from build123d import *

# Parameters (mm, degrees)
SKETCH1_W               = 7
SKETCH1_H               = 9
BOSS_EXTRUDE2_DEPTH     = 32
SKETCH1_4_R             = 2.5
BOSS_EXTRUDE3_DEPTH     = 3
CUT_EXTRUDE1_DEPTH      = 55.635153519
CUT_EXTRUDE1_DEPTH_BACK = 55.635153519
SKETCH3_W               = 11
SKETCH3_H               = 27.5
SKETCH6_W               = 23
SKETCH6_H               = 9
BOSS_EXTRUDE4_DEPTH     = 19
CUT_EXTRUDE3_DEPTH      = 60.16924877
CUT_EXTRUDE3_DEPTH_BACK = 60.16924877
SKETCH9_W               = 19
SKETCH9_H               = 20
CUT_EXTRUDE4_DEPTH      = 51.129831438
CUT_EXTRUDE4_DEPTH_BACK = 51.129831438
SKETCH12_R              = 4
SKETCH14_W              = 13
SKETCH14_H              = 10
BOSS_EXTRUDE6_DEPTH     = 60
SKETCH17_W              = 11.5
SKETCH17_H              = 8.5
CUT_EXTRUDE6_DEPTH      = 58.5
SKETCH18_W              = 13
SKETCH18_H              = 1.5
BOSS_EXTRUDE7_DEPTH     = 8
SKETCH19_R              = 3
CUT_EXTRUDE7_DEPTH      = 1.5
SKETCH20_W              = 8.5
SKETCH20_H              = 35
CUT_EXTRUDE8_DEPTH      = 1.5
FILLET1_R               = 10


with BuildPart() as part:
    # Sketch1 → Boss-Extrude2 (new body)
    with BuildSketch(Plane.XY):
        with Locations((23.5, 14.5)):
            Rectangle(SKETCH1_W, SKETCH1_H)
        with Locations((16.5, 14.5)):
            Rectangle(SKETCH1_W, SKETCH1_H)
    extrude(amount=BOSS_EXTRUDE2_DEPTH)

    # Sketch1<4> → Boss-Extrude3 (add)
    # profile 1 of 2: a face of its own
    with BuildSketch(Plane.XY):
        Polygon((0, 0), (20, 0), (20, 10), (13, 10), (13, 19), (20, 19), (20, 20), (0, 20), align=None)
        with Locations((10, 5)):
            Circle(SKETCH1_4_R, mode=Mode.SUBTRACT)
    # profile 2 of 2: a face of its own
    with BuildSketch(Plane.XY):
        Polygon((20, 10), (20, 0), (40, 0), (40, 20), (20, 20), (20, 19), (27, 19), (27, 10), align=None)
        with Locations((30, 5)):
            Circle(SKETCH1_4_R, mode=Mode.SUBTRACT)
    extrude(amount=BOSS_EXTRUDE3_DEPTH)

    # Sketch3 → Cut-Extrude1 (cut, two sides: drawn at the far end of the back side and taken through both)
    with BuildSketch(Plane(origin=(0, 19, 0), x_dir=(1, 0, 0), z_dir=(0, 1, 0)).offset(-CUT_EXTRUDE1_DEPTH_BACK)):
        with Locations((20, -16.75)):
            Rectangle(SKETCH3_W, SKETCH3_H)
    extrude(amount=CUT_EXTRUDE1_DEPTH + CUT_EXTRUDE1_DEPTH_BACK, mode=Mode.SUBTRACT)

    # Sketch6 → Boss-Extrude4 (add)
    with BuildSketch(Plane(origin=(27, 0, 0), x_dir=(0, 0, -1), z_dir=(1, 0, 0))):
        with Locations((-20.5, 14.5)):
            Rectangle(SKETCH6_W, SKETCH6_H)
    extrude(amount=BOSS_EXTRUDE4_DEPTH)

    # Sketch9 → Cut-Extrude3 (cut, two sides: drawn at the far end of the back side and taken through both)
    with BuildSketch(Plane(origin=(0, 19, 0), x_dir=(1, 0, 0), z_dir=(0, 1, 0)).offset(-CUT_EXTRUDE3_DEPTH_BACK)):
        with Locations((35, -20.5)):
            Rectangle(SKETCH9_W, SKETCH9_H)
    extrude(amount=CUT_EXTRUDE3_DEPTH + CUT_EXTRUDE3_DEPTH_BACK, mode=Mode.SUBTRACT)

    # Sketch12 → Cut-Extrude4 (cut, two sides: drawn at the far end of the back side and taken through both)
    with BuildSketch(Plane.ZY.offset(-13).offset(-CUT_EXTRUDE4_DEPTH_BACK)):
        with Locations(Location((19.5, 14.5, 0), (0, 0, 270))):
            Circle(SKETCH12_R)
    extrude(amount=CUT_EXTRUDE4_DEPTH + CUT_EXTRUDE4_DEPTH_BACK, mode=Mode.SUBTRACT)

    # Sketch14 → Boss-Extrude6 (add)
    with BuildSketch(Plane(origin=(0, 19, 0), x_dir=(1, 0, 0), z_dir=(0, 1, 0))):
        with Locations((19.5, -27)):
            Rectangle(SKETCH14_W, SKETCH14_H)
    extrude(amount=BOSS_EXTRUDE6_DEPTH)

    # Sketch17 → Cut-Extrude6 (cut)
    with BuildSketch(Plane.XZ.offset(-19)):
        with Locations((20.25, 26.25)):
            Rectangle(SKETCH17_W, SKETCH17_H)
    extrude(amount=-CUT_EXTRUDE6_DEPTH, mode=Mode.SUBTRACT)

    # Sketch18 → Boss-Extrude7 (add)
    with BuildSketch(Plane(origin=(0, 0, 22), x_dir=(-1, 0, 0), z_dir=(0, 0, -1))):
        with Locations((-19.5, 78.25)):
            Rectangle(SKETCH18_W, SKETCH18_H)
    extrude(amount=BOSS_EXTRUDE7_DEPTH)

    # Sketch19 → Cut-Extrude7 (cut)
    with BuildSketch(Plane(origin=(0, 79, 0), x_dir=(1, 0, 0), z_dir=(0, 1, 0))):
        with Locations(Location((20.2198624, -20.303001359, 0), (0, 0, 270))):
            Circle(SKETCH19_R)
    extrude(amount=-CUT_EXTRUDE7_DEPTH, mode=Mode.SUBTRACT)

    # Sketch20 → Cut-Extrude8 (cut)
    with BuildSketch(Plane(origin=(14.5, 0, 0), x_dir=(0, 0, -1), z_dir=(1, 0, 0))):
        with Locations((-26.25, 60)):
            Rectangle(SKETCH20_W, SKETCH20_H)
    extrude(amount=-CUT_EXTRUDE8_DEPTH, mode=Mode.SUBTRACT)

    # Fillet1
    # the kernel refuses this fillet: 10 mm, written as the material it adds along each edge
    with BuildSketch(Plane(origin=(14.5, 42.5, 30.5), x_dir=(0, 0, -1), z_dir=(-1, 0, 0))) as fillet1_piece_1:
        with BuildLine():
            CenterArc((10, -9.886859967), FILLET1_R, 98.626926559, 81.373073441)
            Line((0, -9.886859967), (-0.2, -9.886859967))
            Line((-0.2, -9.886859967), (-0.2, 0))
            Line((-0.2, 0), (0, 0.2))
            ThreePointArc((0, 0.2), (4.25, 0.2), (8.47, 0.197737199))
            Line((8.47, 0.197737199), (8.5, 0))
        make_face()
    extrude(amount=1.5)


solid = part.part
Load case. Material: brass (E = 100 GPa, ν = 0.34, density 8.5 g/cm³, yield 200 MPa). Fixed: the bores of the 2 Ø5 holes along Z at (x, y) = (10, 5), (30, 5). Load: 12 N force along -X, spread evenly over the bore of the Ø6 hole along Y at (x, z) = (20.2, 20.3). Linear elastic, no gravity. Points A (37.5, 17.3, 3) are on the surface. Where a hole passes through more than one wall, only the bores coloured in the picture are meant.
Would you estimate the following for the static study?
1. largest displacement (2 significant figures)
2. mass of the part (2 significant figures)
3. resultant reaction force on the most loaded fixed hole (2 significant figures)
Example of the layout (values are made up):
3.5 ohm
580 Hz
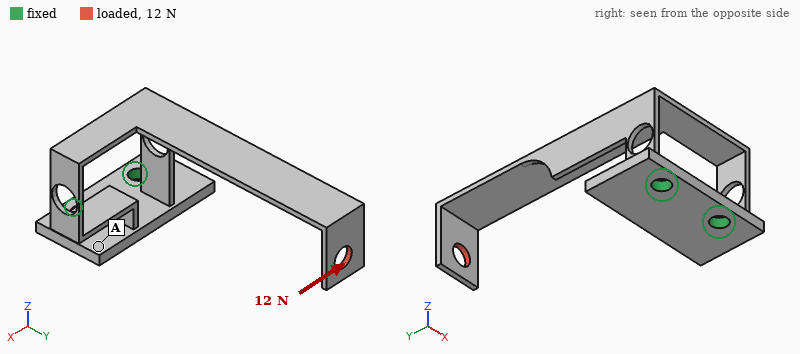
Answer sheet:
1.0 mm
46 g
44 N
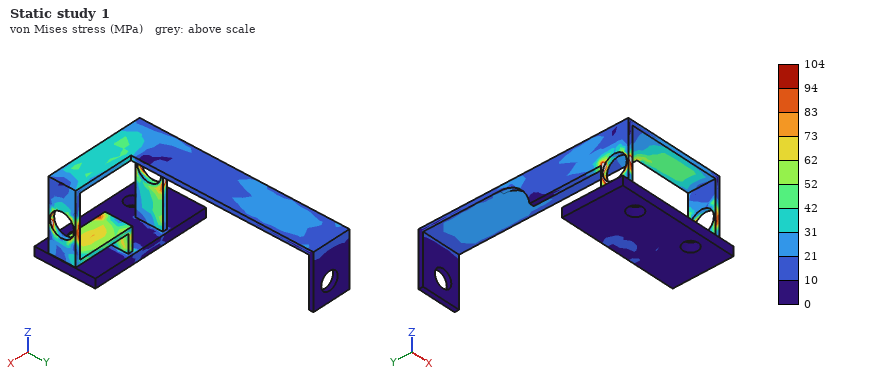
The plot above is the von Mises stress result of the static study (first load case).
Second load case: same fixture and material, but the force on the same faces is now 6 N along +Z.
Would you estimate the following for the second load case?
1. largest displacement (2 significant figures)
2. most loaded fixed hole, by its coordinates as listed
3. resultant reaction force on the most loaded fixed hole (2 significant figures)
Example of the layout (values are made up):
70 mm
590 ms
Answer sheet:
0.44 mm
(30, 5)
5.3 N
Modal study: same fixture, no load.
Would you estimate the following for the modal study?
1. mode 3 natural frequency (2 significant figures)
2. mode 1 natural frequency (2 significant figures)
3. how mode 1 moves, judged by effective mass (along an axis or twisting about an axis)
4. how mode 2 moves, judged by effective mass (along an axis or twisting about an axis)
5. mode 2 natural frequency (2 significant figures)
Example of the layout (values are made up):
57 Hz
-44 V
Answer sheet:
460 Hz
220 Hz
along X
along Z
290 Hz
